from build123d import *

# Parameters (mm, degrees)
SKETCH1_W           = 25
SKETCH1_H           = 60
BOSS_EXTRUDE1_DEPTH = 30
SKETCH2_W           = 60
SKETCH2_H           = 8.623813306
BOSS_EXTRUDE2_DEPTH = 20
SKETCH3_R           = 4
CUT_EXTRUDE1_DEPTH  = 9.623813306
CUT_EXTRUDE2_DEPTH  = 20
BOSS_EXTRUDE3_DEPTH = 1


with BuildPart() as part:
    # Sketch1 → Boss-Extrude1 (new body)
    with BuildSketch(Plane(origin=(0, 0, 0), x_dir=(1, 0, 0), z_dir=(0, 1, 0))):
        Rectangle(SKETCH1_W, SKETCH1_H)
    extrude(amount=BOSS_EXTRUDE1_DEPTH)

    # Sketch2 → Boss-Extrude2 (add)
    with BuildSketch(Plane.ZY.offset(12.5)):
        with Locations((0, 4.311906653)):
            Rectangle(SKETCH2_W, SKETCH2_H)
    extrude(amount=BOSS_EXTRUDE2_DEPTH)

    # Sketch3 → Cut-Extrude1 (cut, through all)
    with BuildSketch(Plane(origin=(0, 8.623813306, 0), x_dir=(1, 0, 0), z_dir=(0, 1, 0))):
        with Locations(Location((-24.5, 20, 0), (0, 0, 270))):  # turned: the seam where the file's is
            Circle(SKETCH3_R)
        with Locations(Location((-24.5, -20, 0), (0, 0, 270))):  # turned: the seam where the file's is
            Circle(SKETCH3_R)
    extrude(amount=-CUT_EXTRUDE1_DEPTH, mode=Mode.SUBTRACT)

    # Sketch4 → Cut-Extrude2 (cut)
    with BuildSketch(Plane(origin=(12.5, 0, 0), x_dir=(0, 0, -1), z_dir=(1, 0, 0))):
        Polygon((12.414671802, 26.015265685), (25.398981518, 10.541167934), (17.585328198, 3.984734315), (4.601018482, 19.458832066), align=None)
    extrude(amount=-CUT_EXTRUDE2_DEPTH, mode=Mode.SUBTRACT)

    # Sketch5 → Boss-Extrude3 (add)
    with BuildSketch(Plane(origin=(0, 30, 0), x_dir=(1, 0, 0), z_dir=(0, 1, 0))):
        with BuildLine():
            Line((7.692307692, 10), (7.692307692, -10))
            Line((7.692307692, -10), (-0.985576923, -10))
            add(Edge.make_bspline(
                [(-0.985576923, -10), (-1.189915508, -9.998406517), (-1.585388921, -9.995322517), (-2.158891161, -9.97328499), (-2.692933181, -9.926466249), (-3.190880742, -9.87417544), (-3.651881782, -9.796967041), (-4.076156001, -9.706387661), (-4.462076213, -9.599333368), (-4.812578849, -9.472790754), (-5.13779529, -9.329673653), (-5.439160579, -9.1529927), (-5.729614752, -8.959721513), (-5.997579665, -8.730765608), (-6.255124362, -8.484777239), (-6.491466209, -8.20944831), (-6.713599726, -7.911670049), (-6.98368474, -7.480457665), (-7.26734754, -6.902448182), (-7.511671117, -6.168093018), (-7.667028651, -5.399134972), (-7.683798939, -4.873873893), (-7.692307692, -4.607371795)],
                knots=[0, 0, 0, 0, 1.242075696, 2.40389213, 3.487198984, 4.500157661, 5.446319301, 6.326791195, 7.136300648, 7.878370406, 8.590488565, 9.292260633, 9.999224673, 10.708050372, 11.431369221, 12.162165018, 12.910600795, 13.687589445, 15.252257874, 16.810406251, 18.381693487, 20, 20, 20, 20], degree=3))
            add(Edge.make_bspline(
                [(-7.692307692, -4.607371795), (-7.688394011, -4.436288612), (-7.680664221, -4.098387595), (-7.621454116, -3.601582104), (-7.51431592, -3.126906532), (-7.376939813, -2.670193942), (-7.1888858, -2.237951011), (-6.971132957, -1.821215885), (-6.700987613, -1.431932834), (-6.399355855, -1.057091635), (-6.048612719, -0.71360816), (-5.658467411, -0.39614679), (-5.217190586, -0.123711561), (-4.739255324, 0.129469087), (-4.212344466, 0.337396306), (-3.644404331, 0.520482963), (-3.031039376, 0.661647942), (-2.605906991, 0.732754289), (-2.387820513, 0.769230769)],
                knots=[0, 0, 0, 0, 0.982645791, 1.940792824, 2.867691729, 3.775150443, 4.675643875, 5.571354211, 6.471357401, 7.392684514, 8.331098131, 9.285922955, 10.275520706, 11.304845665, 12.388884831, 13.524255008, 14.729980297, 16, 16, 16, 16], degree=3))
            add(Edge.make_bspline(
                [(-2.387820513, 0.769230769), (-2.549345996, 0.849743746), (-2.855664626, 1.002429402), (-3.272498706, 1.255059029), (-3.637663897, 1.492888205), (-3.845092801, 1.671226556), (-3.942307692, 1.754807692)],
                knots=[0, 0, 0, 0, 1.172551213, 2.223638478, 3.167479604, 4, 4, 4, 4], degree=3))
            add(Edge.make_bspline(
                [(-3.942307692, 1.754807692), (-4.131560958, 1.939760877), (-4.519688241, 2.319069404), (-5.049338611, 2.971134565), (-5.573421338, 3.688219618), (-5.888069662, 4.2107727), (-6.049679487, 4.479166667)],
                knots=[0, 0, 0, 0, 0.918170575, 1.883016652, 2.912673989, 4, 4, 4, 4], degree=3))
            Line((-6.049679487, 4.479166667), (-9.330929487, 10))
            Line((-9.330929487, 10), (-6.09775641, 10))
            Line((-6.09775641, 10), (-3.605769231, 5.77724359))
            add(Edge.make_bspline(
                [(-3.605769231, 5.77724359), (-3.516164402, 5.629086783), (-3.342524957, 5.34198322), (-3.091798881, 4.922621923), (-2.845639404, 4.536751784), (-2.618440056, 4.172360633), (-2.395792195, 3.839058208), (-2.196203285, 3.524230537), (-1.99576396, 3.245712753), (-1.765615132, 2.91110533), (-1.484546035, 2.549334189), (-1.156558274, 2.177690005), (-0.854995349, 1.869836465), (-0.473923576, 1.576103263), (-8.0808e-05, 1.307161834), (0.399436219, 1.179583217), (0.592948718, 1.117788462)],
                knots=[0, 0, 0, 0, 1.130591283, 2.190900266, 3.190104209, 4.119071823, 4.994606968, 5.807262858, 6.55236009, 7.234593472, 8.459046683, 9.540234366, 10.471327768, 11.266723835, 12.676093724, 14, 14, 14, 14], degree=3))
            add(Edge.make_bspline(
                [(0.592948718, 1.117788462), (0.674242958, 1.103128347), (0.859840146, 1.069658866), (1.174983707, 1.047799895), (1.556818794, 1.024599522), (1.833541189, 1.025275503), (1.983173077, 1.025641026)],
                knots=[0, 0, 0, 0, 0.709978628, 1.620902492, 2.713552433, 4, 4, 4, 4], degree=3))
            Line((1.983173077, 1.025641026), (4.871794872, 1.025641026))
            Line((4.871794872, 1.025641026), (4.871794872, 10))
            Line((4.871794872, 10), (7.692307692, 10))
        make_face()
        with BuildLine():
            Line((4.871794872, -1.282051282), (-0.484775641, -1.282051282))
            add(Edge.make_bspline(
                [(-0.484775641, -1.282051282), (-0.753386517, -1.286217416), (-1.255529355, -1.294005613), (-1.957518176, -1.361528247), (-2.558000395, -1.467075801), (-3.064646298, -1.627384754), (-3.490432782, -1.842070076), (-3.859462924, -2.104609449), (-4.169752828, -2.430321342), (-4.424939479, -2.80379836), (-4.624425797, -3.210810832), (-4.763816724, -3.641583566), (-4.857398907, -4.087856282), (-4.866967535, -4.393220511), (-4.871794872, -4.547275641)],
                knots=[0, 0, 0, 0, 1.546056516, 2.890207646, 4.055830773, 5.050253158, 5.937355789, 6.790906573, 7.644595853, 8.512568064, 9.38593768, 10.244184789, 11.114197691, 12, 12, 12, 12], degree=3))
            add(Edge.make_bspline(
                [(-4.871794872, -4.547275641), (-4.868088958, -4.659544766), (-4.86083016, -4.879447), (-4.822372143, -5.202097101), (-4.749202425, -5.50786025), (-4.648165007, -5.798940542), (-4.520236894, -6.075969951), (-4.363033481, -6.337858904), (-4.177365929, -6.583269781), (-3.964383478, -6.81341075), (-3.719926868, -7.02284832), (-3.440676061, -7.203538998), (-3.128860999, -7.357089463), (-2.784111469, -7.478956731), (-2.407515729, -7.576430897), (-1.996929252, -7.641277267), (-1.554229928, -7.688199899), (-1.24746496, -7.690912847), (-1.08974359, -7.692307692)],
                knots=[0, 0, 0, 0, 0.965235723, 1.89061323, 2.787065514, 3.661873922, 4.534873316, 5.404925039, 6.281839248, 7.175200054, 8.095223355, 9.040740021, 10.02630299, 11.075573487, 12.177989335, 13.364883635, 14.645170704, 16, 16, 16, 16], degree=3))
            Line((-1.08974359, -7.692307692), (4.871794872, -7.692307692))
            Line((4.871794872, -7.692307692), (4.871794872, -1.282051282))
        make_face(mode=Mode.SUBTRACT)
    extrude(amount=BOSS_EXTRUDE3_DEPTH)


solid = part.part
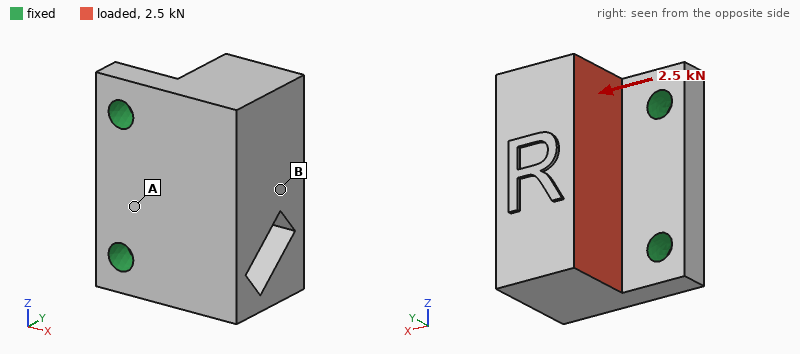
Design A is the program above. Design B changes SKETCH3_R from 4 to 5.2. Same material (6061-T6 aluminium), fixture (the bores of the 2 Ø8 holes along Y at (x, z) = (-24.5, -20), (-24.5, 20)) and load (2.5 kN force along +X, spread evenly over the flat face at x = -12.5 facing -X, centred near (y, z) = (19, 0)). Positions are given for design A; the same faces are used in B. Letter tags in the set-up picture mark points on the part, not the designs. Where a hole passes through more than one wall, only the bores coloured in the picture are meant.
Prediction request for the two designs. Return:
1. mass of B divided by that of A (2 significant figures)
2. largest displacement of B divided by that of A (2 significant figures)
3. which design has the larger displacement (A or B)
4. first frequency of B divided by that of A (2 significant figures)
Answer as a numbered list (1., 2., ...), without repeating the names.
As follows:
1. 0.99
2. 0.87
3. A
4. 1.1
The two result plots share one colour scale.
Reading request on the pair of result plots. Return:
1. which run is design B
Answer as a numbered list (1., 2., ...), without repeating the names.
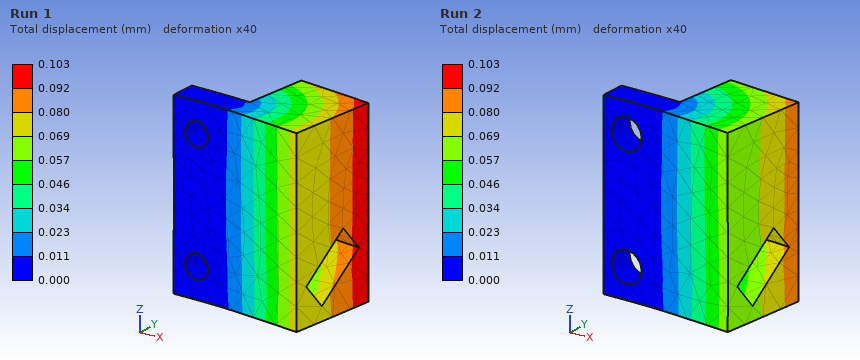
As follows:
1. Run 2
